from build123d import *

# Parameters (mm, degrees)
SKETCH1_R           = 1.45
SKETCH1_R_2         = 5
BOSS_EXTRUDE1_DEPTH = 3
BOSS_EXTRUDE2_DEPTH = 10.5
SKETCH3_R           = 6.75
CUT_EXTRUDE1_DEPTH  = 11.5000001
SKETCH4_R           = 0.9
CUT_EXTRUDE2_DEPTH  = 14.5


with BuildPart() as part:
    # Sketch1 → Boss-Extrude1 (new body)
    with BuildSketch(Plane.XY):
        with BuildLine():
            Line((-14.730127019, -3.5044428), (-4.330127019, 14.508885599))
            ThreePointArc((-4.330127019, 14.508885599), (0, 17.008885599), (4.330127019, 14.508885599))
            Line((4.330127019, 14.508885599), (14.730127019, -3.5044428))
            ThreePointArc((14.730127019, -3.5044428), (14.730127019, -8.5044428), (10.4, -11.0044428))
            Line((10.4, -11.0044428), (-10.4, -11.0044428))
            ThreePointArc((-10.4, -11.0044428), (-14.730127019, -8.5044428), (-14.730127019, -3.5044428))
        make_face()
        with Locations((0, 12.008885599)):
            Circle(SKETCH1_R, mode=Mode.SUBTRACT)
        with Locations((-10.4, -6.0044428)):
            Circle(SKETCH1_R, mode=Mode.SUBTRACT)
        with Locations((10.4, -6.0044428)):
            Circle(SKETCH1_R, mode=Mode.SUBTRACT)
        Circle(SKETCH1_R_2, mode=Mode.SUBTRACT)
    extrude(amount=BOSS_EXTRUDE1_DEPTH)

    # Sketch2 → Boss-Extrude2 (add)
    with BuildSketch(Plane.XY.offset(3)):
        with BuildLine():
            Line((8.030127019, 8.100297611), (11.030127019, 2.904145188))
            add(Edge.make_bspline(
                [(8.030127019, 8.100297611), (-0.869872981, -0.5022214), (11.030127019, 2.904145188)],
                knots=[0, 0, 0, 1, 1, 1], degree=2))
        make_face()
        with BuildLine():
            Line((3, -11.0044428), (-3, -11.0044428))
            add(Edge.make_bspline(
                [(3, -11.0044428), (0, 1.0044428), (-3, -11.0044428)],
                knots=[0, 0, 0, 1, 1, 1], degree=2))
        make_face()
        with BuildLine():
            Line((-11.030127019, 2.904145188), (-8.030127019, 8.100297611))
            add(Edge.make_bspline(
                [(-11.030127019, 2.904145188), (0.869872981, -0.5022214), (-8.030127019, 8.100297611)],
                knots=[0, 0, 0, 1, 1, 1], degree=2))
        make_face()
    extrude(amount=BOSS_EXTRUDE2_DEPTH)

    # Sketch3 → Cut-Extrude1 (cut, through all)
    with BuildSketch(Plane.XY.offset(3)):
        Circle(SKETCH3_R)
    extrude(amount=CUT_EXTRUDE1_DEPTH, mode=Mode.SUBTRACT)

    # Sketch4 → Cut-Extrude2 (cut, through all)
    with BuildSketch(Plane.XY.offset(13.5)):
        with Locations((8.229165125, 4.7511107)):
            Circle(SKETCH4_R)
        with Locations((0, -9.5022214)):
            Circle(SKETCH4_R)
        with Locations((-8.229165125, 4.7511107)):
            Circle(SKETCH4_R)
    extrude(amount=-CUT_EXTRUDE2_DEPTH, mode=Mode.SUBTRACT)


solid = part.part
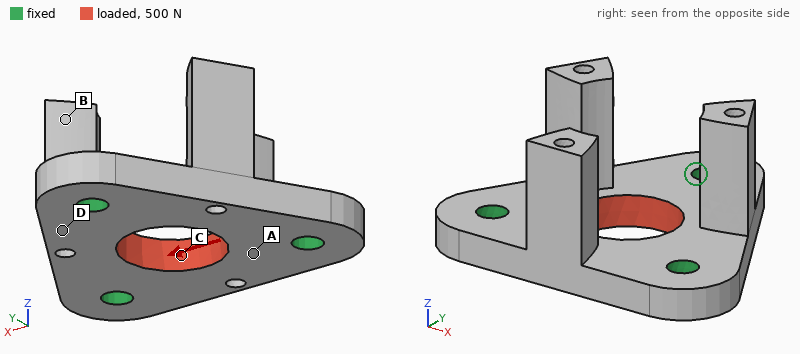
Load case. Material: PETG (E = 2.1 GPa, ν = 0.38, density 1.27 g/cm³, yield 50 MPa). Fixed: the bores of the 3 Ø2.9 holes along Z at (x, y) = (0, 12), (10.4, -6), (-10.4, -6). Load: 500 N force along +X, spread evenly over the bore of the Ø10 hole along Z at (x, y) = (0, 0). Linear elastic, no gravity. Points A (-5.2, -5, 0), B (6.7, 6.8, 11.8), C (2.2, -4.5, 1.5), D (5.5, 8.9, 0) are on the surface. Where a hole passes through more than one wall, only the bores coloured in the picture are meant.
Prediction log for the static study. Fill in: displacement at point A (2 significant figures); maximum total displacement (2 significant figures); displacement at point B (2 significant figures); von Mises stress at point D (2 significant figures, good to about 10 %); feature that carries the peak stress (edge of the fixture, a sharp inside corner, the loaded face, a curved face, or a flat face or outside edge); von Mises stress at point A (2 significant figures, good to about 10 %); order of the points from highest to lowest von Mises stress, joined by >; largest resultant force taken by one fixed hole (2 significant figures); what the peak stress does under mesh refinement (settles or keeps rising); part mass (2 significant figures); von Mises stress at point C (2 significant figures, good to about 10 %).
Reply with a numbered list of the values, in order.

1. 19 µm
2. 84 µm
3. 80 µm
4. 5.2 MPa
5. edge of the fixture
6. 7.7 MPa
7. C > A > D > B
8. 170 N
9. keeps rising
10. 2.5 g
11. 10 MPa
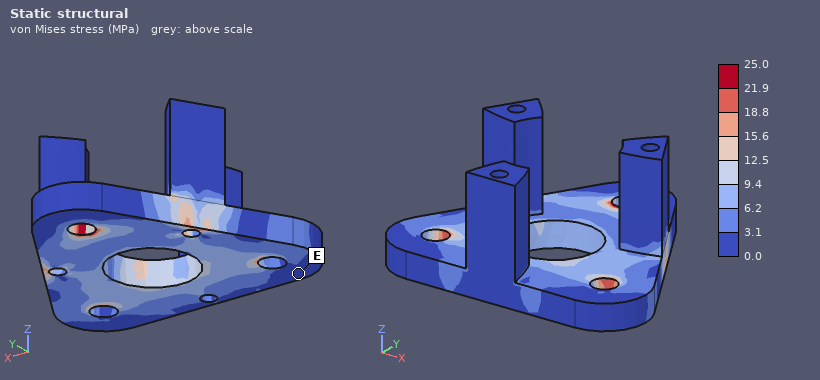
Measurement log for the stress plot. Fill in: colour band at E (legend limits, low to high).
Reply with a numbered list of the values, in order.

1. 0.0 to 3.1 MPa
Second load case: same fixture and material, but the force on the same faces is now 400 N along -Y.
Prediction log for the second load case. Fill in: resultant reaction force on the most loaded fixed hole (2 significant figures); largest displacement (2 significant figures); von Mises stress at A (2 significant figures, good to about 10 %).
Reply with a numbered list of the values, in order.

1. 140 N
2. 77 µm
3. 4.5 MPa
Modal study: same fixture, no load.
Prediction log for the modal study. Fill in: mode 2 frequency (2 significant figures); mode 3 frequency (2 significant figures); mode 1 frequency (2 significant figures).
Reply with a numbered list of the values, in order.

1. 3600 Hz
2. 3600 Hz
3. 3500 Hz
